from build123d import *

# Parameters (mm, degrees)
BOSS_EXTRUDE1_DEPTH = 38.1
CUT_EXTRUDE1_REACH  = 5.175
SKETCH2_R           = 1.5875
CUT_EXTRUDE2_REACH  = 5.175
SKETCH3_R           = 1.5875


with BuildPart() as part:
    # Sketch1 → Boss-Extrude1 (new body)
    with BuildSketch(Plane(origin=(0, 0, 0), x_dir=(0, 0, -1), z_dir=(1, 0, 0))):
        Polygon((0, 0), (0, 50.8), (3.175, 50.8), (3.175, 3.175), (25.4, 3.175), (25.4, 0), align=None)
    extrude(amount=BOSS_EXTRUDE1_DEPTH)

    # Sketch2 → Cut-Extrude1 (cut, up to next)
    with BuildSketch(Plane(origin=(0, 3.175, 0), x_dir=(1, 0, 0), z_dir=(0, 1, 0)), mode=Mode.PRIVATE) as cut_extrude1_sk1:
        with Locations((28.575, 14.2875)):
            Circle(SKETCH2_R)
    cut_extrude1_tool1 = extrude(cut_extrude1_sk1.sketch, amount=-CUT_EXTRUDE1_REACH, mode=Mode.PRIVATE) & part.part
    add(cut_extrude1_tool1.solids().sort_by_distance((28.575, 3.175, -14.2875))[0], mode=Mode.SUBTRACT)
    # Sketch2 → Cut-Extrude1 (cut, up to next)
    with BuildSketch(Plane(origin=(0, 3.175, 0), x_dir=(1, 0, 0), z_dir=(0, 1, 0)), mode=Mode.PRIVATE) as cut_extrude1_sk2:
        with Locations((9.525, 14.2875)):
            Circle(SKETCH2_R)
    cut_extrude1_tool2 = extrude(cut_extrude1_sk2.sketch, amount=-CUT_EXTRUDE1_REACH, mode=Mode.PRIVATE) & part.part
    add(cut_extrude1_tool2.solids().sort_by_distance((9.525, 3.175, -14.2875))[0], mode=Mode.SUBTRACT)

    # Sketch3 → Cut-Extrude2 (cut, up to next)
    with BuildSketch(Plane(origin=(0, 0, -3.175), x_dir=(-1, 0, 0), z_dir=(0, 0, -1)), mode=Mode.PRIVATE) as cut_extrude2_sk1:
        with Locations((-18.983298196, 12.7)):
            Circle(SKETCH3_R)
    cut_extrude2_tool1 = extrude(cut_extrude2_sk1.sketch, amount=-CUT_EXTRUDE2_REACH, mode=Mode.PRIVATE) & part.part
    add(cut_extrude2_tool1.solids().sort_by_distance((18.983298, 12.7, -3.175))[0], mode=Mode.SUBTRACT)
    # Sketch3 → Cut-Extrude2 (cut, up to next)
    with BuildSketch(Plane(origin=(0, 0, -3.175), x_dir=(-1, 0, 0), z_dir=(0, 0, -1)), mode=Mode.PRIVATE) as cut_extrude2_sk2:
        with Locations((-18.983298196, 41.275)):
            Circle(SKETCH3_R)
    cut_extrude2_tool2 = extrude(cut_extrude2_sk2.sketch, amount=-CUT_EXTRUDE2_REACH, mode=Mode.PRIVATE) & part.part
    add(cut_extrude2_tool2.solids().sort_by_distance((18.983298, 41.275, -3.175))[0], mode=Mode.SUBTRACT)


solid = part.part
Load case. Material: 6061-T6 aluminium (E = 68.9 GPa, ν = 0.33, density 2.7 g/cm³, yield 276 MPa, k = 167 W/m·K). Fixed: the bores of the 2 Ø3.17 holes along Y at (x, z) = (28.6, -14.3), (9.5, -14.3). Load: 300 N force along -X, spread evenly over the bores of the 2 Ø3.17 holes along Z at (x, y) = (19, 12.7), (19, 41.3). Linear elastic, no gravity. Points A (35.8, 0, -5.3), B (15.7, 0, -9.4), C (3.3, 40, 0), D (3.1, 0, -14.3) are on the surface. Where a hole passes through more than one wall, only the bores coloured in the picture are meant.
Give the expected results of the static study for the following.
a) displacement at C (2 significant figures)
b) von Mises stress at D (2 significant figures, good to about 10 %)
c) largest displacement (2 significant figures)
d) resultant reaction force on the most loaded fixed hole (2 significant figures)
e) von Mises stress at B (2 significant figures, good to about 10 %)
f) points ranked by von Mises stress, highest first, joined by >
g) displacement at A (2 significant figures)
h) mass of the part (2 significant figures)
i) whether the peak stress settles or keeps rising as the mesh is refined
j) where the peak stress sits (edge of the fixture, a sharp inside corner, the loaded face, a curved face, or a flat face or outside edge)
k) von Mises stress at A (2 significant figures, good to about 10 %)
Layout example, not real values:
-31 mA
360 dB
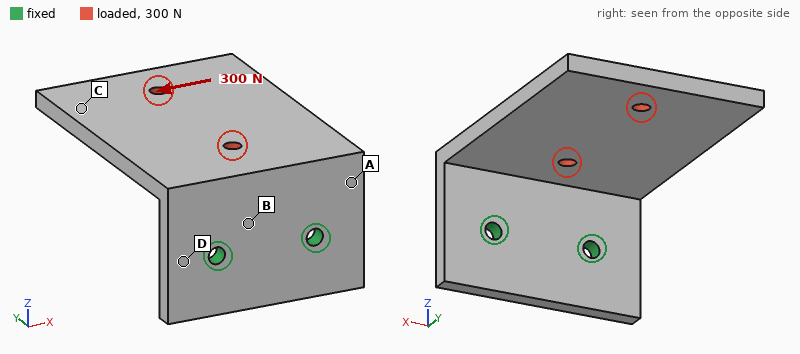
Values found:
0.13 mm
43 MPa
0.17 mm
400 N
31 MPa
D > B > A > C
0.037 mm
24 g
keeps rising
edge of the fixture
21 MPa
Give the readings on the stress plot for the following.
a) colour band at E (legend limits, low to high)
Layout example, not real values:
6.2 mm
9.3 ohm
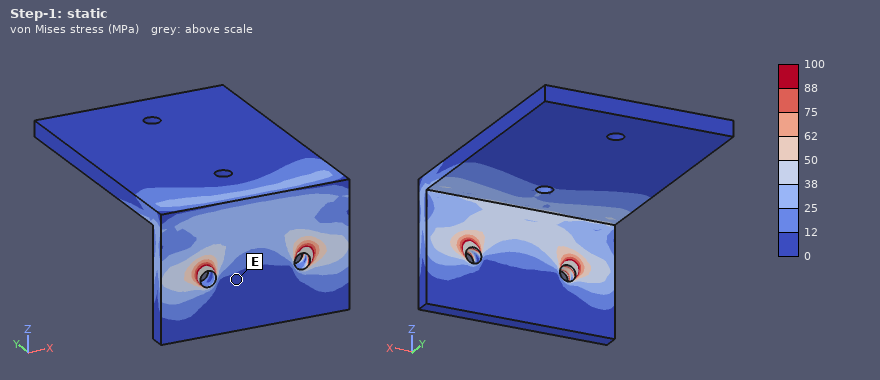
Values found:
0 to 12 MPa
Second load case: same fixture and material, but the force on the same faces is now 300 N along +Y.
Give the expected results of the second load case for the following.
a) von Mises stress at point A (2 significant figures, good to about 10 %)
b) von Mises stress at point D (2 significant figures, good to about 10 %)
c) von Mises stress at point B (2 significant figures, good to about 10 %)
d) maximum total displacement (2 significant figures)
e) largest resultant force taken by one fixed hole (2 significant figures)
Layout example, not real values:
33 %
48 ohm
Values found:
16 MPa
22 MPa
29 MPa
0.18 mm
150 N
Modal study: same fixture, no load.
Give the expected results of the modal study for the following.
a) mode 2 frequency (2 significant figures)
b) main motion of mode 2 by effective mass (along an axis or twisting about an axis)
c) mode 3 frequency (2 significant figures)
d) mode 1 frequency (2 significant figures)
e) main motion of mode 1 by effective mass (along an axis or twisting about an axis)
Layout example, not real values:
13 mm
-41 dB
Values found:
2000 Hz
along X
3100 Hz
770 Hz
along Z
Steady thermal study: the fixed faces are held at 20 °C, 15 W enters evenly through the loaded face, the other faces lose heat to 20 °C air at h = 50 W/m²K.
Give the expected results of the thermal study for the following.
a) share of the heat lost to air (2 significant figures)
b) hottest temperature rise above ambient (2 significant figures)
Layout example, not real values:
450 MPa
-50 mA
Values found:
25 %
25 K
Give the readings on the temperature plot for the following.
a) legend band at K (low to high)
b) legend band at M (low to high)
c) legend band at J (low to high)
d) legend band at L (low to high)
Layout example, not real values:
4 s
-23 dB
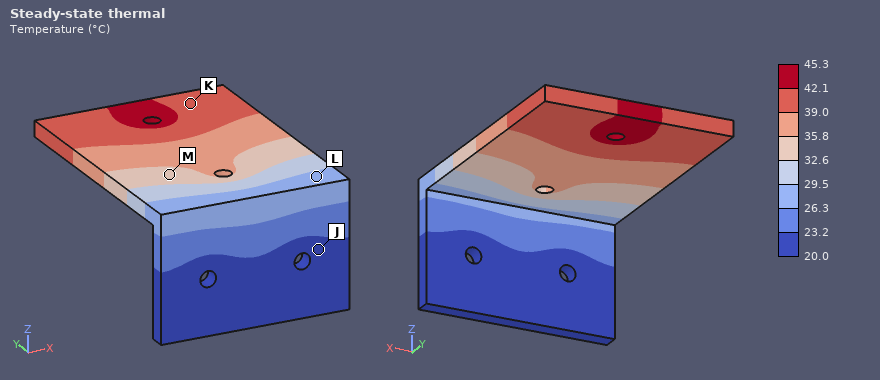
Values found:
39.0 to 42.1 °C
32.6 to 35.8 °C
20.0 to 23.2 °C
26.3 to 29.5 °C
